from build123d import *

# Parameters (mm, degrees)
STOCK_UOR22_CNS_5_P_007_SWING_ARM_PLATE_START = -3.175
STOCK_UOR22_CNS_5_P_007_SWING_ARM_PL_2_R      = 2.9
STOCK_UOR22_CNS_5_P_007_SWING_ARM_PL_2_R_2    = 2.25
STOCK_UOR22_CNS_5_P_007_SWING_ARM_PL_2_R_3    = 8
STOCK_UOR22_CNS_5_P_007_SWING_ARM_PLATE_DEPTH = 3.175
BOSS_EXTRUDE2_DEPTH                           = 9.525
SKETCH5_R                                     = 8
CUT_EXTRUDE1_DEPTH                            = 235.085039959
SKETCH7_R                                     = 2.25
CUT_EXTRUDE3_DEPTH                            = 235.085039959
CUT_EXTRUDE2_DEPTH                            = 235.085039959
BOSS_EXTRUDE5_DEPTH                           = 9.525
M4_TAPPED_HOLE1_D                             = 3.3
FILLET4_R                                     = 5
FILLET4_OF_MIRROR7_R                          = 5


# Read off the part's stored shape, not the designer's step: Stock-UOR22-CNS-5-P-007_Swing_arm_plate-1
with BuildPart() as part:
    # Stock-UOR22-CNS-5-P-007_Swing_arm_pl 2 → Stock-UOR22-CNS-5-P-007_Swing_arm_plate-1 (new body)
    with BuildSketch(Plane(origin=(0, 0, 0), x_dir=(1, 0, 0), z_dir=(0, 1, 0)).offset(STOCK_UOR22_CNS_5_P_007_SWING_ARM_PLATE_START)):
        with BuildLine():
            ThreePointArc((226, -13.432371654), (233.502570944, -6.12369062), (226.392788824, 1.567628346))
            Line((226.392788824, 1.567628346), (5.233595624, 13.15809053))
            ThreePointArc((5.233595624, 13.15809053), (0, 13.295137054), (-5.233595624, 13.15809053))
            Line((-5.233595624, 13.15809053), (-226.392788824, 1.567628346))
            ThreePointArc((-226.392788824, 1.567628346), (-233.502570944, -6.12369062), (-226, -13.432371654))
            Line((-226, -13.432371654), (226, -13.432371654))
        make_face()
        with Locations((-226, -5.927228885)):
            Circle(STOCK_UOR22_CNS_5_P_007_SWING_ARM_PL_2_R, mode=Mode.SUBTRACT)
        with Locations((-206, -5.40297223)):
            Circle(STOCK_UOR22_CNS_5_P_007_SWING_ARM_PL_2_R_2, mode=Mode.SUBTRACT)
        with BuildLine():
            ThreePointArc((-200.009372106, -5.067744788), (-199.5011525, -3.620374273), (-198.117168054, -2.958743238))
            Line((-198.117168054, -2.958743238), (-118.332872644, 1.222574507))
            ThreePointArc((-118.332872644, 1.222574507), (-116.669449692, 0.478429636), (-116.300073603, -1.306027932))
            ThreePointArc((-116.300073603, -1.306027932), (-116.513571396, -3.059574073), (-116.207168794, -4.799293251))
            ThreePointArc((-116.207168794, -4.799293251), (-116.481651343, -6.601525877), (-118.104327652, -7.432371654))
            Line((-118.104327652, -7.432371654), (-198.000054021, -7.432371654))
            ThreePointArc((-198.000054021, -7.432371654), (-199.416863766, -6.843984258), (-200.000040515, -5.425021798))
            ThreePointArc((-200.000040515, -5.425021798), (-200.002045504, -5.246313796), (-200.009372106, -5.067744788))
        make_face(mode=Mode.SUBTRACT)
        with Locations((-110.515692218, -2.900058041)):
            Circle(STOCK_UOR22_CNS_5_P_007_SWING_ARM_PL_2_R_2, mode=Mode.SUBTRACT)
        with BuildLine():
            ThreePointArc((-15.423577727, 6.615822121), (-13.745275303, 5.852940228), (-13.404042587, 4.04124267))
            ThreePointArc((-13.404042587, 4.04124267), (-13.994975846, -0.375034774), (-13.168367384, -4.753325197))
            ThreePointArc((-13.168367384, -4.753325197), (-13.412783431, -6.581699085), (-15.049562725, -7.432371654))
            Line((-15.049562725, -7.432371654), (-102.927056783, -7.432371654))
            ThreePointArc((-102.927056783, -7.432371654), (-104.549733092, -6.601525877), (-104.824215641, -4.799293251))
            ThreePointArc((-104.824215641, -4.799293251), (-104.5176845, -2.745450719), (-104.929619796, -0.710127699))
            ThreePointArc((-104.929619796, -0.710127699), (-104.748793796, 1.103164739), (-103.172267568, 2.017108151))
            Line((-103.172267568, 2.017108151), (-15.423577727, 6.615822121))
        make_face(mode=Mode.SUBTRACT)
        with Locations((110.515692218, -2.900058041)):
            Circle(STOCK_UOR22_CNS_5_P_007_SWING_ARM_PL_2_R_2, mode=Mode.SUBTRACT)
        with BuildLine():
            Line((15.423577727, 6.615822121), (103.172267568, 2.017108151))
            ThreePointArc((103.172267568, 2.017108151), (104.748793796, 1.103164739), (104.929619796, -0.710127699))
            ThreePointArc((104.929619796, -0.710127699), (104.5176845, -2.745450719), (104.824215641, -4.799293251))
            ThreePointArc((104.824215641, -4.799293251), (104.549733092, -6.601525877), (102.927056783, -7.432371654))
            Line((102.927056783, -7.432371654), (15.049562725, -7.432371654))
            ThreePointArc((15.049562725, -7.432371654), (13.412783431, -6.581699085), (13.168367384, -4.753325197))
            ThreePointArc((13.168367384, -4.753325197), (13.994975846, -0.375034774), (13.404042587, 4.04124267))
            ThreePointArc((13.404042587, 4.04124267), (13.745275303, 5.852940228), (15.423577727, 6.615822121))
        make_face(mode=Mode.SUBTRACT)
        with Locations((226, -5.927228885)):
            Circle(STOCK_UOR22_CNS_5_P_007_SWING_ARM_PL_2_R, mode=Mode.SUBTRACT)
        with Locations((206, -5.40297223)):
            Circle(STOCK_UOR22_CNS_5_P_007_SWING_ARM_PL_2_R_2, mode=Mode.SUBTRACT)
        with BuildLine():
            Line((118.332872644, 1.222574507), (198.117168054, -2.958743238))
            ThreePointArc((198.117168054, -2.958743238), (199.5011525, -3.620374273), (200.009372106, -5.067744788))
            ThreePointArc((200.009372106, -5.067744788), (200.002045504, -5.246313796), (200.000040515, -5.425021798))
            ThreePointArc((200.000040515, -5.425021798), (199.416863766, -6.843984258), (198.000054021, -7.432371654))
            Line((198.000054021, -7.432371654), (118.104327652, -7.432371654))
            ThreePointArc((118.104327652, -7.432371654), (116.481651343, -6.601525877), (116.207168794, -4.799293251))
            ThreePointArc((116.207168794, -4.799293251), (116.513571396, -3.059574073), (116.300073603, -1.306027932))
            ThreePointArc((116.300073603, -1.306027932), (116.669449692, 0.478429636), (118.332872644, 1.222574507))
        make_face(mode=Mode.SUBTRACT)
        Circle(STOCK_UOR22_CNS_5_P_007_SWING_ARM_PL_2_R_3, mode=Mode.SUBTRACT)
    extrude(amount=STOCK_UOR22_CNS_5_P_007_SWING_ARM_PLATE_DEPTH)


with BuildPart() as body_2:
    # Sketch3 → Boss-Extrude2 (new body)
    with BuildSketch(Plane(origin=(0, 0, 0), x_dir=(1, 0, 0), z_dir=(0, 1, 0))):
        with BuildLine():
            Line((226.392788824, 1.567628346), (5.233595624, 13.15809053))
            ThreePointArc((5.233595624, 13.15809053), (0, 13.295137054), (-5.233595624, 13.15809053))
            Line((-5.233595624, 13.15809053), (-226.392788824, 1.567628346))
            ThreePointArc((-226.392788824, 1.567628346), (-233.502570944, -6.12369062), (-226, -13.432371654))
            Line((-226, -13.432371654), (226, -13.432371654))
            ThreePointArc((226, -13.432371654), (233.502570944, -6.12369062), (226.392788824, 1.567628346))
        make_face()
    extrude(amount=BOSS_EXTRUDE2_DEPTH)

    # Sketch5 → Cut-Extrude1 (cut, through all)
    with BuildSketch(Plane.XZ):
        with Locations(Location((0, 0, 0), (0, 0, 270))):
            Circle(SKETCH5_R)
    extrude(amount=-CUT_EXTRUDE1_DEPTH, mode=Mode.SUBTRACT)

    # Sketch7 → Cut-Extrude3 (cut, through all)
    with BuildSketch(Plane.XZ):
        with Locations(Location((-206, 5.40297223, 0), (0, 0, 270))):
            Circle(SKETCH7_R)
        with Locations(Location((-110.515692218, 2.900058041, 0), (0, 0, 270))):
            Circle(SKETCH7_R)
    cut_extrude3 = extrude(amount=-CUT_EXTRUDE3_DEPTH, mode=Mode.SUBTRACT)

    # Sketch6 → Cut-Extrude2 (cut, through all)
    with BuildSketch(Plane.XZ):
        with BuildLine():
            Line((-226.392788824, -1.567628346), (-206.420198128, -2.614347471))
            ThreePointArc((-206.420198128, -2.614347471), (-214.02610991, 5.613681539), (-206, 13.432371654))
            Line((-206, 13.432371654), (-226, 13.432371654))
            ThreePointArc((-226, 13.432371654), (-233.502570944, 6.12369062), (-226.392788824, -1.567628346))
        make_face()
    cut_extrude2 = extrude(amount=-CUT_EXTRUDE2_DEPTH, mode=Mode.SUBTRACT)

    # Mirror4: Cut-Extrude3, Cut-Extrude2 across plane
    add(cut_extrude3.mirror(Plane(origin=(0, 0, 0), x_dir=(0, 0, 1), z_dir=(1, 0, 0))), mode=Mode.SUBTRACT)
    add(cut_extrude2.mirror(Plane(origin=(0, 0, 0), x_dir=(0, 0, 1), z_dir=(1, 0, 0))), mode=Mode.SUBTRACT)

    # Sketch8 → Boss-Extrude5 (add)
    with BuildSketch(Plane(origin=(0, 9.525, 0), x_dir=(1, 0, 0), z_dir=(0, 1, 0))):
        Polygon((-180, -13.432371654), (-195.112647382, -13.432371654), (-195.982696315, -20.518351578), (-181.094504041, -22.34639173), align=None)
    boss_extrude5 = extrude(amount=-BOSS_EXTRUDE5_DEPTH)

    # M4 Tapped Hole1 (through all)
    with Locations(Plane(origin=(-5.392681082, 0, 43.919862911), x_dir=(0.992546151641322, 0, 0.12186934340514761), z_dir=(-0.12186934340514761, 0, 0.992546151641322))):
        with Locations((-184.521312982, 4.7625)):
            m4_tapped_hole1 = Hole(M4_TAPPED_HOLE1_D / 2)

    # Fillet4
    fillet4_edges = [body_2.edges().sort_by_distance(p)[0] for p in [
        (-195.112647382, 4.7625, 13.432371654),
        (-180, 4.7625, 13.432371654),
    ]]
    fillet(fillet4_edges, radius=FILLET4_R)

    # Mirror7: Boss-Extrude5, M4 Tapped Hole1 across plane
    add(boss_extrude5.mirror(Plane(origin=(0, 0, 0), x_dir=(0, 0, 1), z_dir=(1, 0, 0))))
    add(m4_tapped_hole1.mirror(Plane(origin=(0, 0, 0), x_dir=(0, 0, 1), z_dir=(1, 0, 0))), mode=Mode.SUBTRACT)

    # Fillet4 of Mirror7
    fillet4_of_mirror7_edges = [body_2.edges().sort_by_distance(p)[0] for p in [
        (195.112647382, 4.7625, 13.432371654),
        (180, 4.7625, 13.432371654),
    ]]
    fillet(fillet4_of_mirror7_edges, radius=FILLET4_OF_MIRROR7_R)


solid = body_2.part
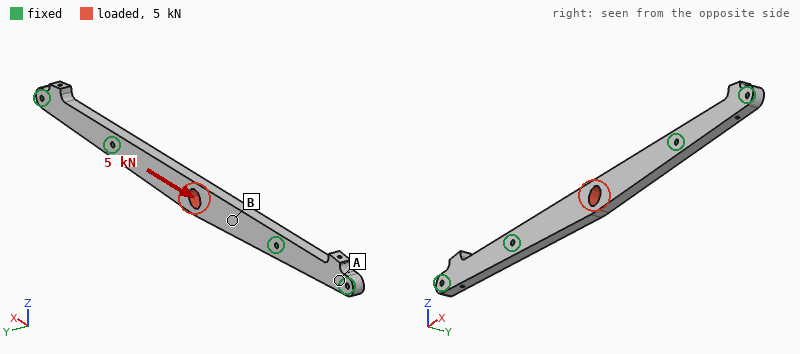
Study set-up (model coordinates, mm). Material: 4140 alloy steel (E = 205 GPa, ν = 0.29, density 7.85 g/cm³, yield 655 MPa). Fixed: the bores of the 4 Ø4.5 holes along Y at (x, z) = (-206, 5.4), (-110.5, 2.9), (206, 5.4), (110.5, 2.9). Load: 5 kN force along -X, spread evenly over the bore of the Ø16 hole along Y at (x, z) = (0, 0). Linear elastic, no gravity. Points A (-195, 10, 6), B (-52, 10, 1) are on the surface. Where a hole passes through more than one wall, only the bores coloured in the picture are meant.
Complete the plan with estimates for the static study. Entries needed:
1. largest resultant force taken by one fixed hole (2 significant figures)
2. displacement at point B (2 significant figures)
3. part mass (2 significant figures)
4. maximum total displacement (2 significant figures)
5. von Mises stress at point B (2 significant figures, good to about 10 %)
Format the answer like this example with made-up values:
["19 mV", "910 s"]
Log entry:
["2.4 kN", "3.6 µm", "670 g", "6.3 µm", "11 MPa"]
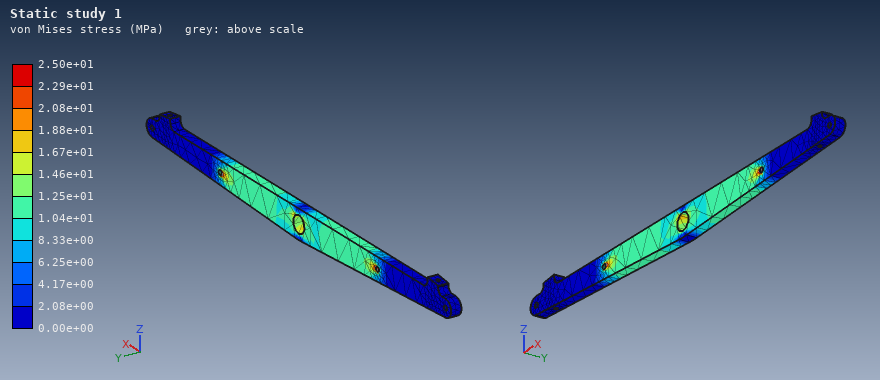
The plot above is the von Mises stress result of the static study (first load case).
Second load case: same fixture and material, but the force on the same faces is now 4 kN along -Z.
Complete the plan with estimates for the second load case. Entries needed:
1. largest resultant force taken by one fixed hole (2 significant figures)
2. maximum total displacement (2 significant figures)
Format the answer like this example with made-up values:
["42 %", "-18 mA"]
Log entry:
["2.8 kN", "0.16 mm"]
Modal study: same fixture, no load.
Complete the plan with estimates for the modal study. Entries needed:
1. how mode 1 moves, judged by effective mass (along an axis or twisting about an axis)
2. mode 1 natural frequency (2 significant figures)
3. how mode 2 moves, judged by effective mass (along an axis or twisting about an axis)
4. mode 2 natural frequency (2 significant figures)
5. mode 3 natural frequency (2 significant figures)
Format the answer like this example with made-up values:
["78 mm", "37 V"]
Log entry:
["along Y", "940 Hz", "along Z", "1900 Hz", "2600 Hz"]
